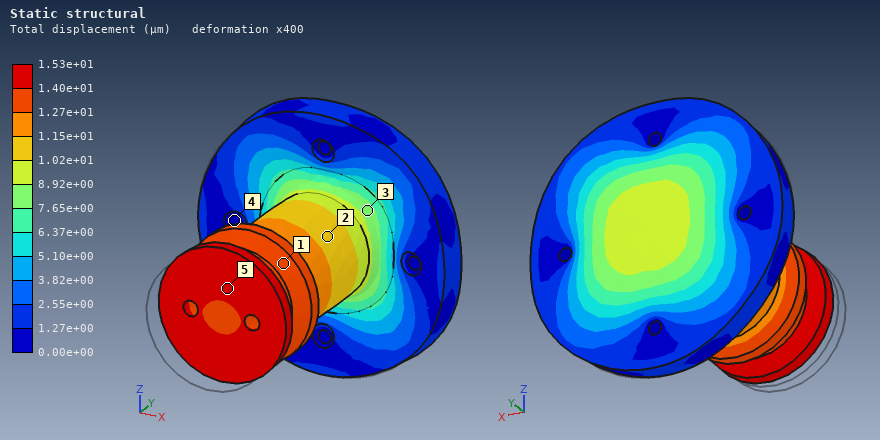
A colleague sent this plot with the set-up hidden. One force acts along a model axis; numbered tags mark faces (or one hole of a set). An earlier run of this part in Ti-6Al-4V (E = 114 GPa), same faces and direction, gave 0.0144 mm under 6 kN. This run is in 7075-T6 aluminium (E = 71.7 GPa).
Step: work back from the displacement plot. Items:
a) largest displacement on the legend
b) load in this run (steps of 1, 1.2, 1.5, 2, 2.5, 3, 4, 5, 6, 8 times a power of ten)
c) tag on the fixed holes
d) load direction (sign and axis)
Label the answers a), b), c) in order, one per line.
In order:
a) 1.53e+01 µm
b) 4 kN
c) 4
d) +Y
